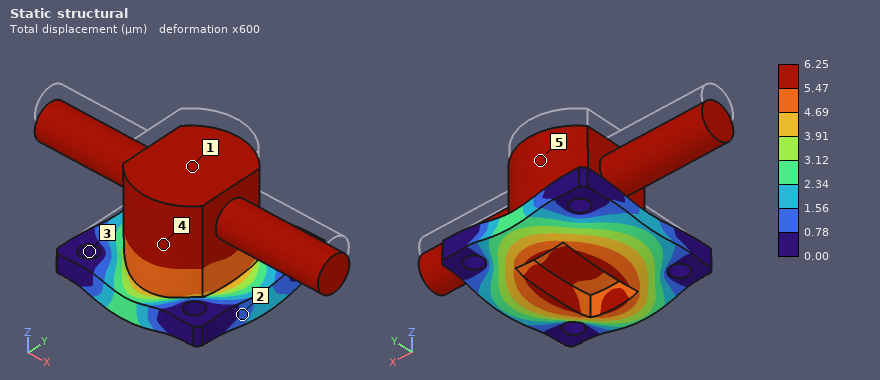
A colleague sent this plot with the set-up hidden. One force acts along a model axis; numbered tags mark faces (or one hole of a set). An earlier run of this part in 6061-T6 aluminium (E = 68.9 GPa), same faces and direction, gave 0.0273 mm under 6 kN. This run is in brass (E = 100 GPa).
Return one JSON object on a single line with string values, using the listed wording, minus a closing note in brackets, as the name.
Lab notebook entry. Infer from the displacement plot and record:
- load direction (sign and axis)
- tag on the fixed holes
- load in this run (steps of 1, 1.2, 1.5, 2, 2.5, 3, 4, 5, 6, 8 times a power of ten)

{"load direction": "-Z", "tag on the fixed holes": "3", "load in this run": "2 kN"}
